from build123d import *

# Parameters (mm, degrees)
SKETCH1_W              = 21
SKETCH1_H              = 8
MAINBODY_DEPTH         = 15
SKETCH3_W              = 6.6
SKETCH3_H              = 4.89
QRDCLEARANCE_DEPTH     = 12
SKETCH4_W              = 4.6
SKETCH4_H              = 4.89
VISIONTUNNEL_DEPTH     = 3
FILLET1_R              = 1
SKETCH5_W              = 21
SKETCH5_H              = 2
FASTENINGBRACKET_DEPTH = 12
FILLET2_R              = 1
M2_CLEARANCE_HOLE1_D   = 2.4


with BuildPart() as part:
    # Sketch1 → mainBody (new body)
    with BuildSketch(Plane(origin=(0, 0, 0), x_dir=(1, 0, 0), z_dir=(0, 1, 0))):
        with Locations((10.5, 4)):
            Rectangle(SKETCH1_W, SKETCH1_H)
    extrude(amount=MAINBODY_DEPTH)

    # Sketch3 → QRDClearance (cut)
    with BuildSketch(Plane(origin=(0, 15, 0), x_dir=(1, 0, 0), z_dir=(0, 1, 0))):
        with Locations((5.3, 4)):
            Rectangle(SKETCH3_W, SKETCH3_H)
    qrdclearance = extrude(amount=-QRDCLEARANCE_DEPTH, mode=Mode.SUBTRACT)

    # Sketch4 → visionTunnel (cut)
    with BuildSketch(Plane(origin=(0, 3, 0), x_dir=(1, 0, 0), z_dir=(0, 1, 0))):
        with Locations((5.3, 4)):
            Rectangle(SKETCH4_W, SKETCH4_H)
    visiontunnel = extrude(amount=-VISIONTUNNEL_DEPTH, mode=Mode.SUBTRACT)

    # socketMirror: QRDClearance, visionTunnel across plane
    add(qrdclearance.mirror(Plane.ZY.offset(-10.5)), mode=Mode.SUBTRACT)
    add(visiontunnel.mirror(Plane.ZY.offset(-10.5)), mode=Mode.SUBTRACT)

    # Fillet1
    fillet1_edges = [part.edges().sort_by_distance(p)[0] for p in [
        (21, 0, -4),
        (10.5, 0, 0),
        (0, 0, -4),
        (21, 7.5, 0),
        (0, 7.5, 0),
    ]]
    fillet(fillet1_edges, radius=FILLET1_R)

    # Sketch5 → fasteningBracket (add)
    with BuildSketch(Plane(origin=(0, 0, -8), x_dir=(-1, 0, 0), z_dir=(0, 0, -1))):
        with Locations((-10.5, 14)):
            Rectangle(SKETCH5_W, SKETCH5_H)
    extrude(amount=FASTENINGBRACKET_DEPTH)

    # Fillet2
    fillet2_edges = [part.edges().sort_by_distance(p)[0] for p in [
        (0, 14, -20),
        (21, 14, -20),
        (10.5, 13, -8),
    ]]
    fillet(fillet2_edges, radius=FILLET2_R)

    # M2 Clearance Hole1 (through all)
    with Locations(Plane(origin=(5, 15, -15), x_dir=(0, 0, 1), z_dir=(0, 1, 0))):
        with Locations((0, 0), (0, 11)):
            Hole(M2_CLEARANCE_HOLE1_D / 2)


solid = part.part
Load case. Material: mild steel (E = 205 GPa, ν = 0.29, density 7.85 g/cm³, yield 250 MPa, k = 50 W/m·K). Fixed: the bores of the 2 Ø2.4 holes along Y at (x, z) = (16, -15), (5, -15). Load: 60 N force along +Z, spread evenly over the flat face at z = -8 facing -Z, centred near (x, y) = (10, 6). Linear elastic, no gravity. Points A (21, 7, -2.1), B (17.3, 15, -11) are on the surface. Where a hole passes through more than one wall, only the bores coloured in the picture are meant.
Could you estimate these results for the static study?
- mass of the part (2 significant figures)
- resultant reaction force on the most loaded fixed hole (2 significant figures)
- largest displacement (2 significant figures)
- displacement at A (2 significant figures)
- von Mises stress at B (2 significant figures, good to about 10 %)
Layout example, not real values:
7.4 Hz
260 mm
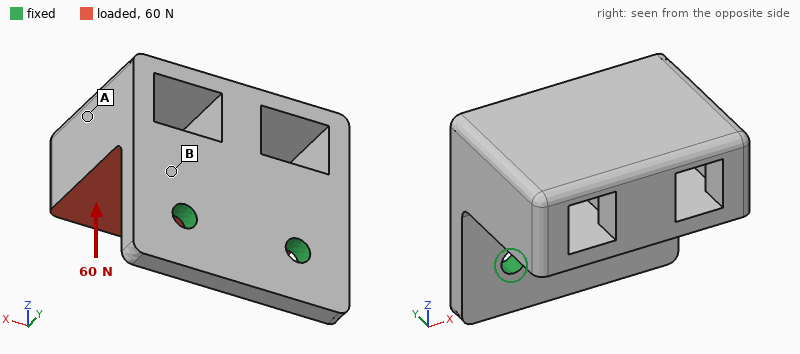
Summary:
16 g
30 N
22 µm
14 µm
30 MPa
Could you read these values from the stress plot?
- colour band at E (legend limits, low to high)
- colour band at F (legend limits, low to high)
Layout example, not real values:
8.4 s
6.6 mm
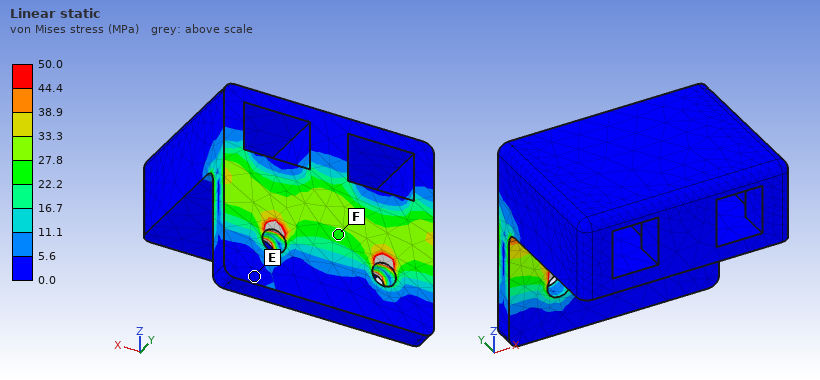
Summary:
0.0 to 5.6 MPa
22.2 to 27.8 MPa
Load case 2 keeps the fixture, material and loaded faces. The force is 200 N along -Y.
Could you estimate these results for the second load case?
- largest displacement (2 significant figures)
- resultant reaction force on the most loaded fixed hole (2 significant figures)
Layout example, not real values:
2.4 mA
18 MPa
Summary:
28 µm
100 N
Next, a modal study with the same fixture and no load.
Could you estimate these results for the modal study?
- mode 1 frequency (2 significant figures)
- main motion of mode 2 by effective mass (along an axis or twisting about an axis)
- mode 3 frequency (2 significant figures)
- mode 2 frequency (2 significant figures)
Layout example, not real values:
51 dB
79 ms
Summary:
2500 Hz
along X
13 kHz
6400 Hz
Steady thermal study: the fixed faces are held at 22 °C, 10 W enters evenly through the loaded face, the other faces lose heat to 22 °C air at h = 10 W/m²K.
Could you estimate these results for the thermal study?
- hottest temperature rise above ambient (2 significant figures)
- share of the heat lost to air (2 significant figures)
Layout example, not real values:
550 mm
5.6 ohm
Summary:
58 K
7.6 %
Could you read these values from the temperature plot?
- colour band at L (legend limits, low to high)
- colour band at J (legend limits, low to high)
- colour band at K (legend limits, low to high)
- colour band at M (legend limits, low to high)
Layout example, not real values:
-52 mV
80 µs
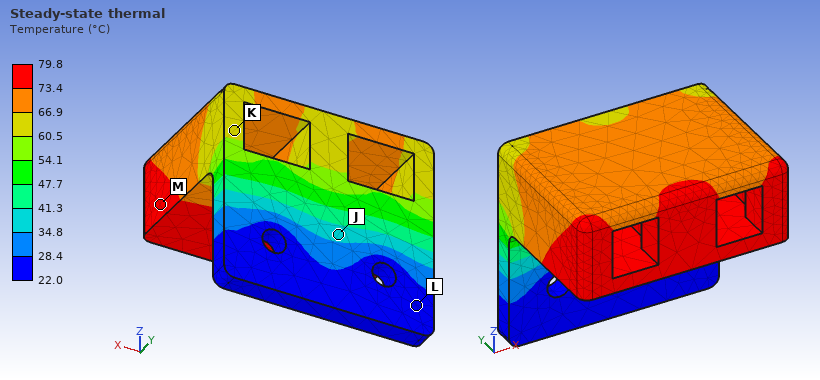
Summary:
22.0 to 28.4 °C
34.8 to 41.3 °C
60.5 to 66.9 °C
73.4 to 79.8 °C
